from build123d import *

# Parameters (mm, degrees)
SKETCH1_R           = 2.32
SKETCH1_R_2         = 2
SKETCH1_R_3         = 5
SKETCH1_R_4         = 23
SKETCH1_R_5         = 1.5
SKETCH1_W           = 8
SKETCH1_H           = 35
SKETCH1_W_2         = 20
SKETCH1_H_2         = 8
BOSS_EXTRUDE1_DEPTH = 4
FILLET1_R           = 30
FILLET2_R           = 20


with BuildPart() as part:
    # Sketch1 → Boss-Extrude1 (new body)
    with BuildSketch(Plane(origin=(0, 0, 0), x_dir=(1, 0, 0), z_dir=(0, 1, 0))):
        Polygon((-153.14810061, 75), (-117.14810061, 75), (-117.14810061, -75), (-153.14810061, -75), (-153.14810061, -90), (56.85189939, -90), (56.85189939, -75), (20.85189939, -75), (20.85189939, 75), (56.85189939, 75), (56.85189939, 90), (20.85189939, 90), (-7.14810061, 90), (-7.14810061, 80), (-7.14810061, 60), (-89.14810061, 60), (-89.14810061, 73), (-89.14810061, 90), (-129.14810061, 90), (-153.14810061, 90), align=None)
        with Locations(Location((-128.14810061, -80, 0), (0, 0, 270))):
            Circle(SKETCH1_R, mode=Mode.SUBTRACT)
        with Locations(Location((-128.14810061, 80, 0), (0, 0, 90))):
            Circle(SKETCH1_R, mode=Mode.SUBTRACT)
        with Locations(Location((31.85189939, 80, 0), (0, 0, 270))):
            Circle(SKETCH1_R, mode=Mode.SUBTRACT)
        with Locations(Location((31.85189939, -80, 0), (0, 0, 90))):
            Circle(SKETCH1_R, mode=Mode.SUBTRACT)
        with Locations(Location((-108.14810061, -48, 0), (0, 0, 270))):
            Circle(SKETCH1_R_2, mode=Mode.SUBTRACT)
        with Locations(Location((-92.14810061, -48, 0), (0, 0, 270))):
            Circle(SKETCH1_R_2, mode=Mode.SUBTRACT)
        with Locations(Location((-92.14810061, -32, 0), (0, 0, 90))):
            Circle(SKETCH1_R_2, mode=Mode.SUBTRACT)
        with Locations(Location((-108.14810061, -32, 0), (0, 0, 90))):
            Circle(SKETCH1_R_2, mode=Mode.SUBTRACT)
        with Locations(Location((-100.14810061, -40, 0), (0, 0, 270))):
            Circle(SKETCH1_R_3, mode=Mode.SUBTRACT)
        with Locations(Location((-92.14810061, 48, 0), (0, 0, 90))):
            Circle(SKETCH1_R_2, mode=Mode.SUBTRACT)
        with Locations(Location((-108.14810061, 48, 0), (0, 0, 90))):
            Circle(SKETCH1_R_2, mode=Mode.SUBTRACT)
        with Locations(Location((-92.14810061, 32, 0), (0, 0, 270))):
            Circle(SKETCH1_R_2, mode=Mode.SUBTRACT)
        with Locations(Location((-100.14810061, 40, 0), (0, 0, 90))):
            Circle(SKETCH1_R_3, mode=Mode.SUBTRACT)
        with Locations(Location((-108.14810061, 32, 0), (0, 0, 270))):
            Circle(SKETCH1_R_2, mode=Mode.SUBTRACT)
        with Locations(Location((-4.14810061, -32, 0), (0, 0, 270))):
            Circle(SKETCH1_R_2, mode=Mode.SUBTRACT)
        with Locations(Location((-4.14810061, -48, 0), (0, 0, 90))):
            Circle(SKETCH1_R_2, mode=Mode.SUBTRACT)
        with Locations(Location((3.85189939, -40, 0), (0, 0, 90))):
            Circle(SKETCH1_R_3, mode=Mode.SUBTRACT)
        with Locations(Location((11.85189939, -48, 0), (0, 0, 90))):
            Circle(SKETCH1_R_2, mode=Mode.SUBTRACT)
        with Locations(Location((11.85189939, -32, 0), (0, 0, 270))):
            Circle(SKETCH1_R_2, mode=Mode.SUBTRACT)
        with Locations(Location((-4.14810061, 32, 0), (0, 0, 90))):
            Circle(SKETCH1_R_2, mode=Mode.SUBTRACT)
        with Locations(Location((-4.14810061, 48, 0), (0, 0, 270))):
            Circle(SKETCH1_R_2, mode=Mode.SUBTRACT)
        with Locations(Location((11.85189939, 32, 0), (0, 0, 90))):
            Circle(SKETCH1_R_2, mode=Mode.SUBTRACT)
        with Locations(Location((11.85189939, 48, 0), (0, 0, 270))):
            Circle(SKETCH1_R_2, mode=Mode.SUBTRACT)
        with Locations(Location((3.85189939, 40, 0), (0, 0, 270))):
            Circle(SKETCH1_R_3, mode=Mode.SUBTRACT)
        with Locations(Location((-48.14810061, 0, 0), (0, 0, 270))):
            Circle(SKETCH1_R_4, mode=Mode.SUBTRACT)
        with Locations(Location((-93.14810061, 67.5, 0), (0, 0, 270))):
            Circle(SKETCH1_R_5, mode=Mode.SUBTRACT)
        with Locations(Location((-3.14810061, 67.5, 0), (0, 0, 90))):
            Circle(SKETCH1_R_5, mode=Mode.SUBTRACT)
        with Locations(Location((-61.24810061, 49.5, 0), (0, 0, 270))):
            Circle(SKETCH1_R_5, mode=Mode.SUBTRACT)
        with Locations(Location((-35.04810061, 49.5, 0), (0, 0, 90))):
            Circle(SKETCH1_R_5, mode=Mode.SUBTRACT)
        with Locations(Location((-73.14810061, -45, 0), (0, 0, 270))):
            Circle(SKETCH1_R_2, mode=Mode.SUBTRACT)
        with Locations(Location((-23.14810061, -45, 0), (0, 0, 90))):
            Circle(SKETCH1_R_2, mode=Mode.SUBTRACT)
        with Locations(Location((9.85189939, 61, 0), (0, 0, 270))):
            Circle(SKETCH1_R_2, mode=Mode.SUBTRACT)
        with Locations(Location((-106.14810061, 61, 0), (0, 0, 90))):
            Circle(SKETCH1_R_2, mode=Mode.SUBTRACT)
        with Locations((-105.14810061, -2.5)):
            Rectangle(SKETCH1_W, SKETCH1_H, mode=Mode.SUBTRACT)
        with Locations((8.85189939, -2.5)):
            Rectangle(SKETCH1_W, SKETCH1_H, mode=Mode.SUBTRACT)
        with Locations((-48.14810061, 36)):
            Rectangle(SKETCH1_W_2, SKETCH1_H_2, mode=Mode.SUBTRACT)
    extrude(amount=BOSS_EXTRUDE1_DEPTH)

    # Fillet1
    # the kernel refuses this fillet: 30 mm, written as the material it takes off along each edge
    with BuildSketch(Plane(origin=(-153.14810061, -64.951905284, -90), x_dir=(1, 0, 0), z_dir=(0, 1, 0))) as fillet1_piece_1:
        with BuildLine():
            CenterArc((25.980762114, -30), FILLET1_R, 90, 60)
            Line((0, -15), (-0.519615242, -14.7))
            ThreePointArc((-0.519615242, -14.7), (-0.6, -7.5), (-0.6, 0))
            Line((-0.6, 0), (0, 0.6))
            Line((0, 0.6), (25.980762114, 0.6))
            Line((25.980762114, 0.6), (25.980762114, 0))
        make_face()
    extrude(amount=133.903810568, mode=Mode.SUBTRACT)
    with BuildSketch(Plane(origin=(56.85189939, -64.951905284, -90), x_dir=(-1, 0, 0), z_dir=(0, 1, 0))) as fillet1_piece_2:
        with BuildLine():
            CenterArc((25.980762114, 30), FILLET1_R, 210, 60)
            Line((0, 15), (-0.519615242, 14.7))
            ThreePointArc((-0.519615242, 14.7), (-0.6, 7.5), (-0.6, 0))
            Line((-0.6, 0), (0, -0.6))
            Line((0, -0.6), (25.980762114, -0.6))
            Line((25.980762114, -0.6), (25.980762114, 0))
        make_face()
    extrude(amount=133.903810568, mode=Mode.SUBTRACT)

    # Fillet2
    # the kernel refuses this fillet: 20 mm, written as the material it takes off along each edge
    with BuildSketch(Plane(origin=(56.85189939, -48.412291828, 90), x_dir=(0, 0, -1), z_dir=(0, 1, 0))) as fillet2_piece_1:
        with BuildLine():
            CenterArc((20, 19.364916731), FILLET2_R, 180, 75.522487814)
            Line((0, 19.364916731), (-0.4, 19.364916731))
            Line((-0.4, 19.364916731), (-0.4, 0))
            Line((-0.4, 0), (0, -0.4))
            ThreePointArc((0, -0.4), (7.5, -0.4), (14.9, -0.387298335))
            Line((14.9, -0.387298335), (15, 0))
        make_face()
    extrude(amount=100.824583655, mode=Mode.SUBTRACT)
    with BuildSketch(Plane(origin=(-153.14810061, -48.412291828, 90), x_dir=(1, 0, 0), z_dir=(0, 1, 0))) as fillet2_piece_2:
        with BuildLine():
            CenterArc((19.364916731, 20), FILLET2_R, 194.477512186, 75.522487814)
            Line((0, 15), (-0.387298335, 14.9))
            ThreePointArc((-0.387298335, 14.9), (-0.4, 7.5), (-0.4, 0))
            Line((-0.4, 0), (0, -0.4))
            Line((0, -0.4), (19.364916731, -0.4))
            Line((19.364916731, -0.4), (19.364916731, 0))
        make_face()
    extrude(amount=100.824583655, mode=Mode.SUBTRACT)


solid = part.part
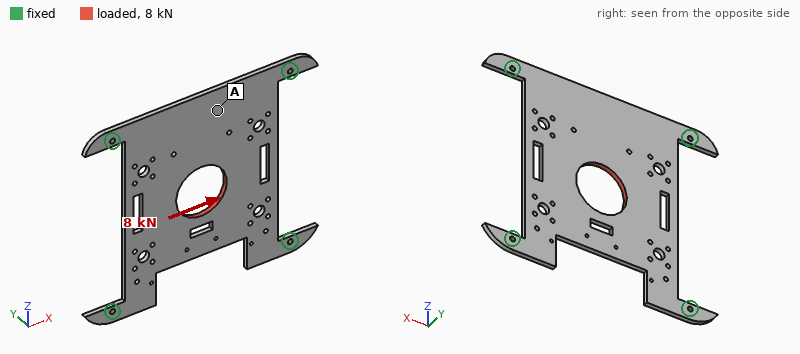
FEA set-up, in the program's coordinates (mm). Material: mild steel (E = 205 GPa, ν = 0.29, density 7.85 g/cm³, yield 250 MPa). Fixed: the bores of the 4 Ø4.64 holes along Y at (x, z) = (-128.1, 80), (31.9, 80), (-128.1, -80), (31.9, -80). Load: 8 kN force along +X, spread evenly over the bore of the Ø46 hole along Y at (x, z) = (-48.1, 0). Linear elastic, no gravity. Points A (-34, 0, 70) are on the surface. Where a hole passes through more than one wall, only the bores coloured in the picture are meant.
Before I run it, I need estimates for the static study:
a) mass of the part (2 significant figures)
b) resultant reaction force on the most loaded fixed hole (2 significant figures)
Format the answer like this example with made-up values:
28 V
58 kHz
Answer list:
660 g
2.5 kN
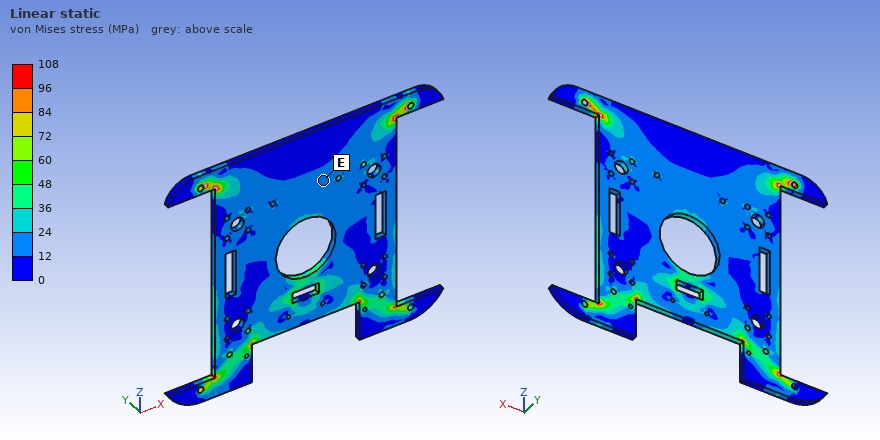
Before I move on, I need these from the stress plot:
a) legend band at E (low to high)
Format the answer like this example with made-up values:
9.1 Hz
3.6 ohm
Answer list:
12 to 24 MPa
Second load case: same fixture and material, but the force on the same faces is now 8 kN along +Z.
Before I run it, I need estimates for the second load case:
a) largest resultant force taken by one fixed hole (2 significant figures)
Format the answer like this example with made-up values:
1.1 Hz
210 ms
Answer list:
2.4 kN
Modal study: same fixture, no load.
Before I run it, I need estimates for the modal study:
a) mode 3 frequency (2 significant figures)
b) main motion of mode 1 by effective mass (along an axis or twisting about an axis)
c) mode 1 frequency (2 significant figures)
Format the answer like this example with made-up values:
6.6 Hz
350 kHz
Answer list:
810 Hz
along Y
400 Hz
